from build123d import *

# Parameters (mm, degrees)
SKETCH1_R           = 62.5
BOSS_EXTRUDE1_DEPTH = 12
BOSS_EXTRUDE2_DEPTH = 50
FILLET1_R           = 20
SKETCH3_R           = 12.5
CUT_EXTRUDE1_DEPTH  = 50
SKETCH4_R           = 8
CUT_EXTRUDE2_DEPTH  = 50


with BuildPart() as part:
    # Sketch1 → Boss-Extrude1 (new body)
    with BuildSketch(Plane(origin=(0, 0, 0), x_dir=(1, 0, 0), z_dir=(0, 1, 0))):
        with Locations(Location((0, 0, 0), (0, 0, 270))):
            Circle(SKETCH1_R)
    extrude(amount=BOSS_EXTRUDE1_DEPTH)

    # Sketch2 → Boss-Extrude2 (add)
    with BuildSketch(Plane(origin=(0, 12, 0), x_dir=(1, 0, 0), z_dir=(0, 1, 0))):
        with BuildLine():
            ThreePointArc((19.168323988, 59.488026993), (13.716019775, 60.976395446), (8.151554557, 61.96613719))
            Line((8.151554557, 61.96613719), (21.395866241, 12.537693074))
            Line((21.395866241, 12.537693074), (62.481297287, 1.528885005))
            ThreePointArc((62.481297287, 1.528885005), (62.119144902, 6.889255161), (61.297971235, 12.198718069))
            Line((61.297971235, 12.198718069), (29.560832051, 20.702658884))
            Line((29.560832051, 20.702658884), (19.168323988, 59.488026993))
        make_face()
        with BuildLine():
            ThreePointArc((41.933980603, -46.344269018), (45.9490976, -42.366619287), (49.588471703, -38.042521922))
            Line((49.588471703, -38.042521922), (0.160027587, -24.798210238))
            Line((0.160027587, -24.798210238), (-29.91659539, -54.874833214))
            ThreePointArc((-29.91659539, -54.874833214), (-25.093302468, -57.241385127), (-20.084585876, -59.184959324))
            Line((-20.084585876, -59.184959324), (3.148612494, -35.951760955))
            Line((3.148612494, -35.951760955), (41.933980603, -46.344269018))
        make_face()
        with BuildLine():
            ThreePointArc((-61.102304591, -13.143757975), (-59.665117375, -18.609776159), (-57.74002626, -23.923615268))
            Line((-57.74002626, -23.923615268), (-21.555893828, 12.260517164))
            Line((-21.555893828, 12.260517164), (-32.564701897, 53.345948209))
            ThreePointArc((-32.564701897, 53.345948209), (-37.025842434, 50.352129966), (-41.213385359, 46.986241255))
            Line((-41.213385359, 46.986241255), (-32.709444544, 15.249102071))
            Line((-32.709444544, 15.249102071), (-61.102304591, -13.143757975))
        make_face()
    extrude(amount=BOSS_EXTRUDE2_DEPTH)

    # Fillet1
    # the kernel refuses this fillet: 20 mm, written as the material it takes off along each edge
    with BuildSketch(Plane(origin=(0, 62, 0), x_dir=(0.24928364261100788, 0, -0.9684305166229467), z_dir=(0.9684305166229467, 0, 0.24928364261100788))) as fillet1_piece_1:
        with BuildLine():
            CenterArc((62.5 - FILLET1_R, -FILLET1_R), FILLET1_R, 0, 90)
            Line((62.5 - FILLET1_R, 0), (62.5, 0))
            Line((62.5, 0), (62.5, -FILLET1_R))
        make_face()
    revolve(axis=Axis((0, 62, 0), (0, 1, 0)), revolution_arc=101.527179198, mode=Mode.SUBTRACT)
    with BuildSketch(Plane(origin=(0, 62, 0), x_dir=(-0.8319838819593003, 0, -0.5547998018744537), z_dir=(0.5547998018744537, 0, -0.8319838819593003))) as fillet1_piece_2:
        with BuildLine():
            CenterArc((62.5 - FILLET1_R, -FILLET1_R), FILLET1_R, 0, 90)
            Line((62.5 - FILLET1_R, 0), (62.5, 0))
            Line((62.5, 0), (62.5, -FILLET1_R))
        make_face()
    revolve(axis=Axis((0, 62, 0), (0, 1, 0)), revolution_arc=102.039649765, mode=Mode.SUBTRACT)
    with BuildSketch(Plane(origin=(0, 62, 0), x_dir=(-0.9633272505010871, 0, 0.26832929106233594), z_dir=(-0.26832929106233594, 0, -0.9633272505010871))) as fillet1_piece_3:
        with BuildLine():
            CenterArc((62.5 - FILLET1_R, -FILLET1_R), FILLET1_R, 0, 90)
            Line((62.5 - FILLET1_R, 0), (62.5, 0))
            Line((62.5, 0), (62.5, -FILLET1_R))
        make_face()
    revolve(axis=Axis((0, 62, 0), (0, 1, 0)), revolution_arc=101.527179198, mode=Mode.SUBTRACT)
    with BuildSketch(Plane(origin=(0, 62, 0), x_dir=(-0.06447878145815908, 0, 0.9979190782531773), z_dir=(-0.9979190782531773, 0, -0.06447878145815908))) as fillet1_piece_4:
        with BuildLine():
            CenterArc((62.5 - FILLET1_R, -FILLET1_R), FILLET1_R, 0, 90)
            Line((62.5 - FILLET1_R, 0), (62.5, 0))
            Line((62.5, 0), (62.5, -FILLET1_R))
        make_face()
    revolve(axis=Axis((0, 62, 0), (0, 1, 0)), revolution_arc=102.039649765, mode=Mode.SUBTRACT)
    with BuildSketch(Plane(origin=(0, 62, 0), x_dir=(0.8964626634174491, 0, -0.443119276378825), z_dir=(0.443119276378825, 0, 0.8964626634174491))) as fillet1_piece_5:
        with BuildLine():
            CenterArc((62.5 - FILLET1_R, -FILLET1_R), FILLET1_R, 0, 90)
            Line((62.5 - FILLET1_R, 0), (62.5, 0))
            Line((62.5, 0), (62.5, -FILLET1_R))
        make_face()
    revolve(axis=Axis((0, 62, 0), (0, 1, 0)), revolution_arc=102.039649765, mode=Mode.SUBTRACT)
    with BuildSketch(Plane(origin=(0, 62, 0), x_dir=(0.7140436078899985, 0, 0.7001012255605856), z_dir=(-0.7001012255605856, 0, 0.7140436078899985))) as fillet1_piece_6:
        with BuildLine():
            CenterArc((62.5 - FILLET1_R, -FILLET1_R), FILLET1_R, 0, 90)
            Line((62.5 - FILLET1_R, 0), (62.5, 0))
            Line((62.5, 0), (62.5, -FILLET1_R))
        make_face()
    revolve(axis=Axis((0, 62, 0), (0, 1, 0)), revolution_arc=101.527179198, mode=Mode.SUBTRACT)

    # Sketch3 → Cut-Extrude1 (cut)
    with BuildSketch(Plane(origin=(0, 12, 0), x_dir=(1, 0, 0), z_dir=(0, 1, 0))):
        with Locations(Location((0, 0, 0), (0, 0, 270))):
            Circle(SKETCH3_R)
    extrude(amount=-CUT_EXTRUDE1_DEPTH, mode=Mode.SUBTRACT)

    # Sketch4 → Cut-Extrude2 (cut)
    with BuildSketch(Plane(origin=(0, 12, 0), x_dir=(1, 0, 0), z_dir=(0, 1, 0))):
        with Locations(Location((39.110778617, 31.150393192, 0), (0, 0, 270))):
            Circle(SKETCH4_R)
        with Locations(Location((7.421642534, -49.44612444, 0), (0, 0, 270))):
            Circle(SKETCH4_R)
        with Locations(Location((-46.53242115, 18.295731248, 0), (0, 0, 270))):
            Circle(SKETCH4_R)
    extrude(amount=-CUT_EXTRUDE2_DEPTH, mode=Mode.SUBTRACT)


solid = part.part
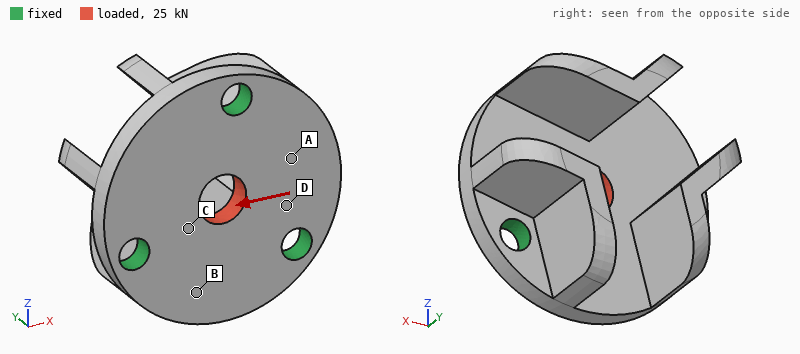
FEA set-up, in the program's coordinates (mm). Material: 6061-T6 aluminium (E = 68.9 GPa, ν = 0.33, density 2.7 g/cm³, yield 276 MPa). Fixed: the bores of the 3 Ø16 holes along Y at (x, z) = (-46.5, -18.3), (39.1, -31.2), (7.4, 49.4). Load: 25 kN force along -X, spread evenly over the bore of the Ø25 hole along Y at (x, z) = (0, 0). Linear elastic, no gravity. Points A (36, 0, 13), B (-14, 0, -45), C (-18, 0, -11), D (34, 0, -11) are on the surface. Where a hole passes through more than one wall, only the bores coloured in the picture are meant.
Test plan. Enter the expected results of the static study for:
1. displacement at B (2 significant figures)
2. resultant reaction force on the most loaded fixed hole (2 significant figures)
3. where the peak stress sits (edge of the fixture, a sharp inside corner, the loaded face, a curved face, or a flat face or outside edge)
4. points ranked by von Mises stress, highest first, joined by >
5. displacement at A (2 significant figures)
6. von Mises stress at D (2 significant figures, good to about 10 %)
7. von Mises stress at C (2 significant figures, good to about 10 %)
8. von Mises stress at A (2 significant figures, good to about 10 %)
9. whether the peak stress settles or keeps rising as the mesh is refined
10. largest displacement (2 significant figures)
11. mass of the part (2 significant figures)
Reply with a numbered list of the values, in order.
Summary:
1. 3.6 µm
2. 8.9 kN
3. edge of the fixture
4. C > D > A > B
5. 12 µm
6. 18 MPa
7. 27 MPa
8. 10 MPa
9. keeps rising
10. 19 µm
11. 690 g
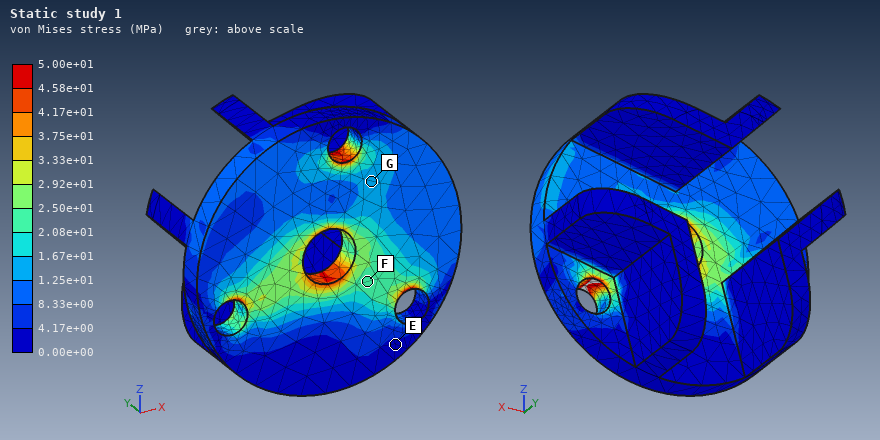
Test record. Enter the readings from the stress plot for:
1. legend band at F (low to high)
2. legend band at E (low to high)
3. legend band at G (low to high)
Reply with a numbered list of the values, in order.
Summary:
1. 2.08e+01 to 2.50e+01 MPa
2. 0.00e+00 to 4.17e+00 MPa
3. 1.25e+01 to 1.67e+01 MPa
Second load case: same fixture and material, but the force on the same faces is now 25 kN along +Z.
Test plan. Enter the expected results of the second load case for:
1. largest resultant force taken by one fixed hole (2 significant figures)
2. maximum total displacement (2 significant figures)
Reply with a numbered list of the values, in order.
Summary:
1. 9.1 kN
2. 19 µm
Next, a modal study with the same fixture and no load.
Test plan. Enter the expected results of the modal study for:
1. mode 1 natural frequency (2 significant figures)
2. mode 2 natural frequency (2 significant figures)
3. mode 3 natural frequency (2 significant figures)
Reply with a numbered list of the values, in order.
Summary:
1. 3200 Hz
2. 3700 Hz
3. 3700 Hz
